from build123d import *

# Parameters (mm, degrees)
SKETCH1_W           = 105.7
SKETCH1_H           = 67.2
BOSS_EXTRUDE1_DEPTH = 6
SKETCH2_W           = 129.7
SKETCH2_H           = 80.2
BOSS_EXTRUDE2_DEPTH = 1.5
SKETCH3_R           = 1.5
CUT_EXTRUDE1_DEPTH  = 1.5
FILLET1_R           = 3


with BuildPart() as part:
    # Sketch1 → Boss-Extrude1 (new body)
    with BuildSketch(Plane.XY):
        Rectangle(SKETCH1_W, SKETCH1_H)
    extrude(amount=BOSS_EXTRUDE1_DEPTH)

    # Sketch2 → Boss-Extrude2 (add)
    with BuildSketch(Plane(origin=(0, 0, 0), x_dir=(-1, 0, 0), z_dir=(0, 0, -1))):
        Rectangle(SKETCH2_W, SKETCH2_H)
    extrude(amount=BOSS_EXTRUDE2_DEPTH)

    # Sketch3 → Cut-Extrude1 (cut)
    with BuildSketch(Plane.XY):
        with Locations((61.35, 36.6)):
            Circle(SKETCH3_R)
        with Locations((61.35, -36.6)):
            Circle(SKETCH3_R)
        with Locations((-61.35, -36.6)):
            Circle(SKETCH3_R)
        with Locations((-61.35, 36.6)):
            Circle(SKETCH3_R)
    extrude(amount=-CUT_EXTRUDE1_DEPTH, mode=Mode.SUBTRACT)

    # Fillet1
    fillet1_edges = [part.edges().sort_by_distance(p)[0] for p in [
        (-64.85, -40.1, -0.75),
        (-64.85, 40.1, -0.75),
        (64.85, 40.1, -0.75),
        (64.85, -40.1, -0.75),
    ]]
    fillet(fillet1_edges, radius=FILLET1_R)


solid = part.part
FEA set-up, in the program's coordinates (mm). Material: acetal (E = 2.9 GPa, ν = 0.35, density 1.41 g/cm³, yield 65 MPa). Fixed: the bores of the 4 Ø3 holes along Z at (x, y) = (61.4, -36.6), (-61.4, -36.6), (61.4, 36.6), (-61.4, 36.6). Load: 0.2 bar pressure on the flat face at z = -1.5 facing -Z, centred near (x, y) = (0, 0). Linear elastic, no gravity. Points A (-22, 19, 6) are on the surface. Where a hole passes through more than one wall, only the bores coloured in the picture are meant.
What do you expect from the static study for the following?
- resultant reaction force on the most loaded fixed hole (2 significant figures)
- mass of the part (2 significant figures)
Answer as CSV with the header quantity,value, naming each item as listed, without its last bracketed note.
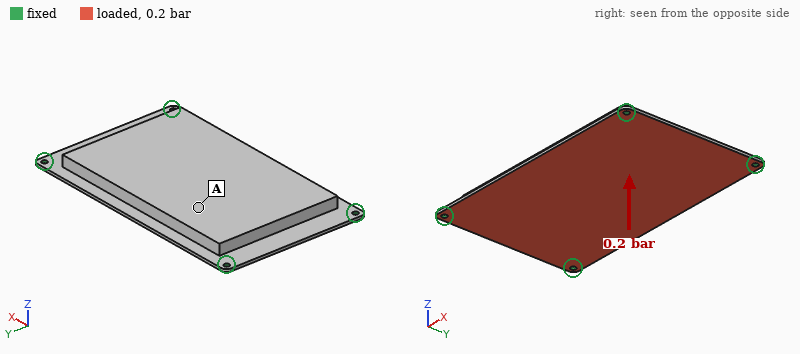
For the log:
quantity,value
resultant reaction force on the most loaded fixed hole,110 N
mass of the part,82 g
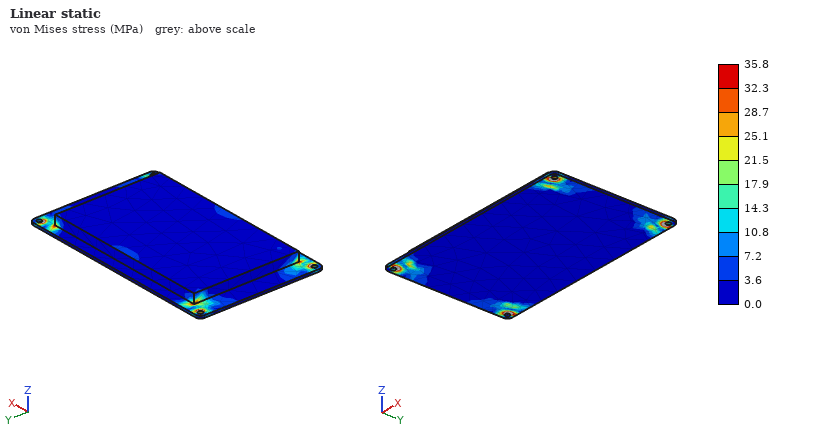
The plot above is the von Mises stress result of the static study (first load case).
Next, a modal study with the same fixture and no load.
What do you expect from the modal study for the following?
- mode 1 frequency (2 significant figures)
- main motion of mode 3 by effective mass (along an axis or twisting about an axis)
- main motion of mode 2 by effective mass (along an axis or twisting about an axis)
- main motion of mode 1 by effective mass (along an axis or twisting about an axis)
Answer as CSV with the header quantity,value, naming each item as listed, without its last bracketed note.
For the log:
quantity,value
mode 1 frequency,290 Hz
main motion of mode 3 by effective mass,twisting about Y
main motion of mode 2 by effective mass,twisting about X
main motion of mode 1 by effective mass,along Z
